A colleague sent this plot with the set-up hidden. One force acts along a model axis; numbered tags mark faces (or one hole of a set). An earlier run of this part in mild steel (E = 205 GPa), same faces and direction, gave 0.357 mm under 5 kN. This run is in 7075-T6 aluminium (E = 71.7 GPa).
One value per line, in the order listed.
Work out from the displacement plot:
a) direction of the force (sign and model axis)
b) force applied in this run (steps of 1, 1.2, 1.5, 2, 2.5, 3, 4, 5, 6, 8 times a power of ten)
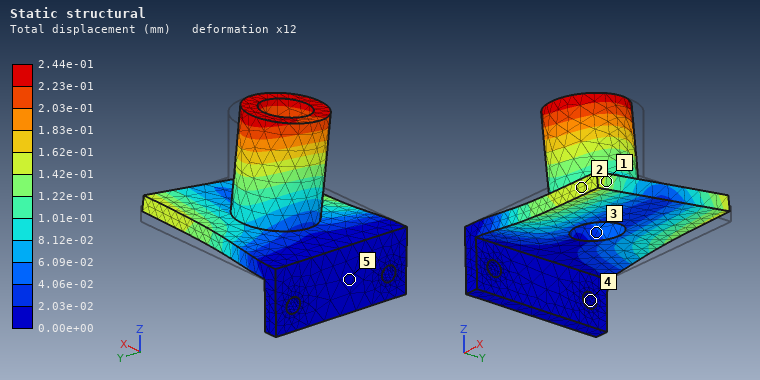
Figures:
-Y
1.2 kN
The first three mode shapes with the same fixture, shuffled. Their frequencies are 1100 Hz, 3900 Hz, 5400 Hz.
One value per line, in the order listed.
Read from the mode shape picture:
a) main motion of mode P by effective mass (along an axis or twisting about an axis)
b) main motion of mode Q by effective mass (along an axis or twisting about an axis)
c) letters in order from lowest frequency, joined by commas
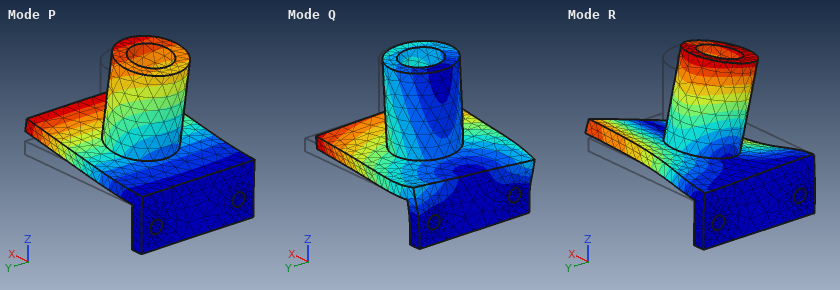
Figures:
along Z
along Y
P, R, Q
